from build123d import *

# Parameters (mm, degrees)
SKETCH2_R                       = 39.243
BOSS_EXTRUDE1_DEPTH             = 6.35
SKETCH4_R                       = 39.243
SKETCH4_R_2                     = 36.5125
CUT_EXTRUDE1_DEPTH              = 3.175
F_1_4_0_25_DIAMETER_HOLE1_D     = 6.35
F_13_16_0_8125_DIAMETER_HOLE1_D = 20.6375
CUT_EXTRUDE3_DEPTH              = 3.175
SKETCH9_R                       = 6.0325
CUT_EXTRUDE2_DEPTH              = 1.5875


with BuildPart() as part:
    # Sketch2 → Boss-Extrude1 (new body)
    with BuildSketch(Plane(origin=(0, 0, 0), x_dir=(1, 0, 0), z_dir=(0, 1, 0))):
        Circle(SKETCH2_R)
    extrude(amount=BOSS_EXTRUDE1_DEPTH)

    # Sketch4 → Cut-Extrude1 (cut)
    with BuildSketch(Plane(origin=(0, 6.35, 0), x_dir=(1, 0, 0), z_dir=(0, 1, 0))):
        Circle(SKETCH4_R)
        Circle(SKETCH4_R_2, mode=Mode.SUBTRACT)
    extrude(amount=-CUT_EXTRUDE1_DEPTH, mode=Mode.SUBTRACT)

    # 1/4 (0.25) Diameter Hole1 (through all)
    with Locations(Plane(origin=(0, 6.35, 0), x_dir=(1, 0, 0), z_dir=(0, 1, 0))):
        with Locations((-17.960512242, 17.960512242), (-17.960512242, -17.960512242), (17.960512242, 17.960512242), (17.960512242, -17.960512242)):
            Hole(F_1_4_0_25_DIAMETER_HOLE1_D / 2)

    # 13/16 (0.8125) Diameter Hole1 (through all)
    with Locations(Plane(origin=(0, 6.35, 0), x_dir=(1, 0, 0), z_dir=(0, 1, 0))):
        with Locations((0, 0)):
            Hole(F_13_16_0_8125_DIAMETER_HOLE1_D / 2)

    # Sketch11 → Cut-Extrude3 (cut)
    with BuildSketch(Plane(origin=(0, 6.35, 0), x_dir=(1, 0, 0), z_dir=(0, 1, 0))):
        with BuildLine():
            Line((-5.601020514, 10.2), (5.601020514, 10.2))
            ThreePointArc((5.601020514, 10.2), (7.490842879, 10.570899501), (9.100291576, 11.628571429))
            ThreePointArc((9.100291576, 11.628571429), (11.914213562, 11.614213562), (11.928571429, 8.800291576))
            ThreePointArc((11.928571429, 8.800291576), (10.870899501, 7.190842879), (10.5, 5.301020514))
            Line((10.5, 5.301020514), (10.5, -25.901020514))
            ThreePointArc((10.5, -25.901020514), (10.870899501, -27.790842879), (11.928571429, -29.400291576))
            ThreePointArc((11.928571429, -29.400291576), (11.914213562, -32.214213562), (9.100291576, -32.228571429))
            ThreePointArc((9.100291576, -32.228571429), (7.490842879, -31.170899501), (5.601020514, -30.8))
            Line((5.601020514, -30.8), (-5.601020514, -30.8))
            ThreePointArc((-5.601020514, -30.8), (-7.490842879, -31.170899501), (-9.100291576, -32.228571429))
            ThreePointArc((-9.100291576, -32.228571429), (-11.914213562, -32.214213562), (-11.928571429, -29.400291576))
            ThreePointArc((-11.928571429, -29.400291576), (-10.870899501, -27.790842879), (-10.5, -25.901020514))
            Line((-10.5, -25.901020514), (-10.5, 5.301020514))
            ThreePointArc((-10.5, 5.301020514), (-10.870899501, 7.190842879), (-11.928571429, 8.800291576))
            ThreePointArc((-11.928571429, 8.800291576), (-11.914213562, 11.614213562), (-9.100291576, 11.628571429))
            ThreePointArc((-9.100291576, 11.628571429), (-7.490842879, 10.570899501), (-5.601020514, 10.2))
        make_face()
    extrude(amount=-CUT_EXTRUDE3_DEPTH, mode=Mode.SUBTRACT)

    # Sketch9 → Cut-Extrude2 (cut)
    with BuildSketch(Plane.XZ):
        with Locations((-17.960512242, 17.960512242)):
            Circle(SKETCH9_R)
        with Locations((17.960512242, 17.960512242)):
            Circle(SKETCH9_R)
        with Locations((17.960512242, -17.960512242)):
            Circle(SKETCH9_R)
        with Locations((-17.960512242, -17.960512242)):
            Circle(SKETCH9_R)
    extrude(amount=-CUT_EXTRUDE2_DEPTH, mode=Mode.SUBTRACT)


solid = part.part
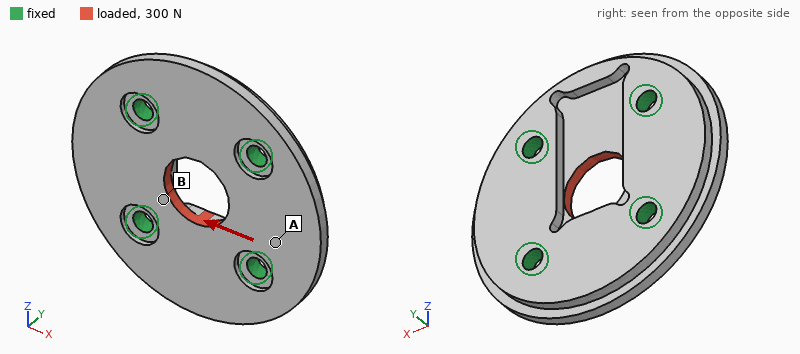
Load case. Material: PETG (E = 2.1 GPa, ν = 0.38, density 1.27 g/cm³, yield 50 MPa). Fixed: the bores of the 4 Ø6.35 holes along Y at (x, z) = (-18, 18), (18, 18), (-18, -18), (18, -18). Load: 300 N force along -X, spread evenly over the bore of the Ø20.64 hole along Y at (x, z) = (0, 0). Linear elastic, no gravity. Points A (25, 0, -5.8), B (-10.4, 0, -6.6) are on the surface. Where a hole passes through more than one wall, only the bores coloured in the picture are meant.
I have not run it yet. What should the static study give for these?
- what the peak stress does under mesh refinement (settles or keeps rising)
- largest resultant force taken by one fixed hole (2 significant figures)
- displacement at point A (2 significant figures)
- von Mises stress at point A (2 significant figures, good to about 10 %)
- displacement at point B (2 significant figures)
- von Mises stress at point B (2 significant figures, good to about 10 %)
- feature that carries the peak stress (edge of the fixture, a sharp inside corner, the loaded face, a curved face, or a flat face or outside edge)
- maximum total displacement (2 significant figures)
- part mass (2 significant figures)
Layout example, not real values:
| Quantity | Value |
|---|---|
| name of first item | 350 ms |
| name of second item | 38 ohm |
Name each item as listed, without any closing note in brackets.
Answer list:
| Quantity | Value |
|---|---|
| what the peak stress does under mesh refinement | keeps rising |
| largest resultant force taken by one fixed hole | 83 N |
| displacement at point A | 8.3 µm |
| von Mises stress at point A | 0.48 MPa |
| displacement at point B | 13 µm |
| von Mises stress at point B | 1.4 MPa |
| feature that carries the peak stress | edge of the fixture |
| maximum total displacement | 20 µm |
| part mass | 30 g |
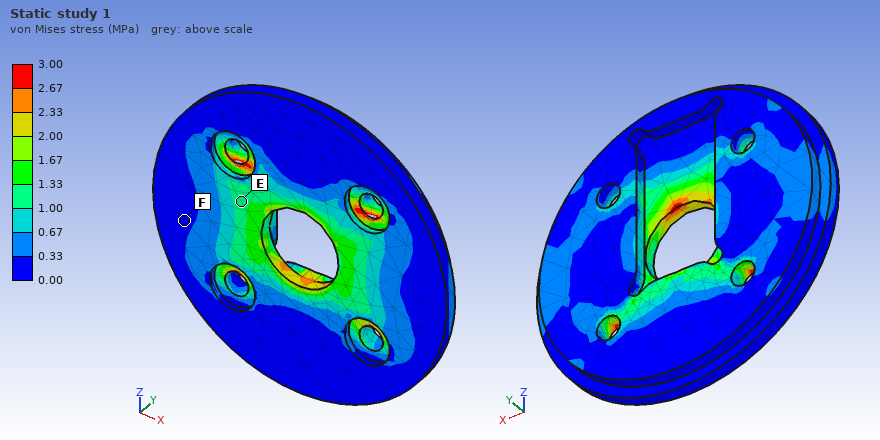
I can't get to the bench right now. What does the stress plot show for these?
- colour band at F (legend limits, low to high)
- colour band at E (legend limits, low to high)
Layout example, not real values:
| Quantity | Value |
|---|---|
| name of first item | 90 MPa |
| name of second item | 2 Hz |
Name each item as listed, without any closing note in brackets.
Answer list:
| Quantity | Value |
|---|---|
| colour band at F | 0.00 to 0.33 MPa |
| colour band at E | 1.00 to 1.33 MPa |
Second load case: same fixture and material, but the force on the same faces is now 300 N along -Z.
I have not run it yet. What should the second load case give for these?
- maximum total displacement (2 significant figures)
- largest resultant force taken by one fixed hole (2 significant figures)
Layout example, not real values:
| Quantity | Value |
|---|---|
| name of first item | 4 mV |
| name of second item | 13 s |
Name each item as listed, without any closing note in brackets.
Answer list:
| Quantity | Value |
|---|---|
| maximum total displacement | 16 µm |
| largest resultant force taken by one fixed hole | 80 N |
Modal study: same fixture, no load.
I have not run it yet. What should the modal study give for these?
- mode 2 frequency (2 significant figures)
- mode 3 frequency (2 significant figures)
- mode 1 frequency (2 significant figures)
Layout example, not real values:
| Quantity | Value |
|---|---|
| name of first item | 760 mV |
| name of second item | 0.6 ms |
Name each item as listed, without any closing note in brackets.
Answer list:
| Quantity | Value |
|---|---|
| mode 2 frequency | 2800 Hz |
| mode 3 frequency | 2800 Hz |
| mode 1 frequency | 2600 Hz |
